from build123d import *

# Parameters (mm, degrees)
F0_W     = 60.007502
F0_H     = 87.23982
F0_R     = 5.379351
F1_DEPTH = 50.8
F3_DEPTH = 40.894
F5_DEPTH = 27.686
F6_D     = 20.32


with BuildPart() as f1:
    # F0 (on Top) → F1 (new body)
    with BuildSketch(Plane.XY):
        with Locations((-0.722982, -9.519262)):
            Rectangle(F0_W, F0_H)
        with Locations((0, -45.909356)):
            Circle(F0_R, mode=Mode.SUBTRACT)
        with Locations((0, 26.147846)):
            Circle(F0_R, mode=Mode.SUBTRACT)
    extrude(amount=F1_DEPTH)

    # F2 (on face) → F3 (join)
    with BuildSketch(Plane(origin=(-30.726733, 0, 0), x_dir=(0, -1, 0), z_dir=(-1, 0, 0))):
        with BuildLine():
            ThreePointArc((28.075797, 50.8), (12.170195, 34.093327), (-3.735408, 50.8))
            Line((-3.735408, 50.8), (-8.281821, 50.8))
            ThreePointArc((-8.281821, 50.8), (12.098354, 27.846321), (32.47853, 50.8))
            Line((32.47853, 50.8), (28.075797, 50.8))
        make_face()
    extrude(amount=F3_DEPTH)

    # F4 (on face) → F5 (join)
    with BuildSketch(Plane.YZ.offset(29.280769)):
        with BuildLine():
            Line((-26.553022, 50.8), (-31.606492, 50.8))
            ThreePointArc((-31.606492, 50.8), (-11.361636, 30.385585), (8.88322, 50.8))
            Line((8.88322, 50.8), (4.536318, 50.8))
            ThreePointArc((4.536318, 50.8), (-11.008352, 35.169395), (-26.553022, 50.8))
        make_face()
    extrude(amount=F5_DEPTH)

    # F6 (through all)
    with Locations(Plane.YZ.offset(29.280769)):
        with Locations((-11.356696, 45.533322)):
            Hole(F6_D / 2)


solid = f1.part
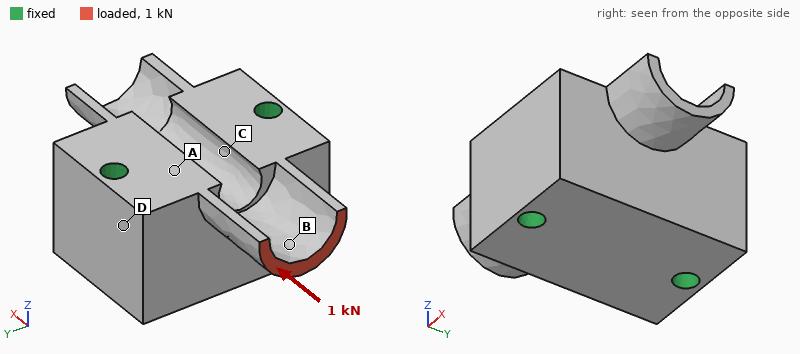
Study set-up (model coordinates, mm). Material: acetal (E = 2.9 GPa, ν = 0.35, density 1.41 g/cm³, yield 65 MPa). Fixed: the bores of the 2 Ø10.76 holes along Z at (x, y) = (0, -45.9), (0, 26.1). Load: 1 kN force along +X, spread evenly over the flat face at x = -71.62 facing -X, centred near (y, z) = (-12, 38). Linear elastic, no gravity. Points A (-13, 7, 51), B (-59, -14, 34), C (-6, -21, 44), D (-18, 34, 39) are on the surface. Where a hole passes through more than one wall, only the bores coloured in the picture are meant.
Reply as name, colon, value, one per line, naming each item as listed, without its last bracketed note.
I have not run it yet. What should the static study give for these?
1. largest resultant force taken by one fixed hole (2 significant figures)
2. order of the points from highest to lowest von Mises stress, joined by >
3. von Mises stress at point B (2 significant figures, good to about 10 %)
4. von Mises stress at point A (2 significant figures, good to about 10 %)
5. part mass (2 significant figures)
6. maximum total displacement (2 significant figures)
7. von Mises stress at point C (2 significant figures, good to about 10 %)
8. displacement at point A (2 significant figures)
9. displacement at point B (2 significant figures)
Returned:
largest resultant force taken by one fixed hole: 550 N
order of the points from highest to lowest von Mises stress, joined by >: B > A > C > D
von Mises stress at point B: 3.0 MPa
von Mises stress at point A: 0.97 MPa
part mass: 370 g
maximum total displacement: 61 µm
von Mises stress at point C: 0.53 MPa
displacement at point A: 9.9 µm
displacement at point B: 43 µm
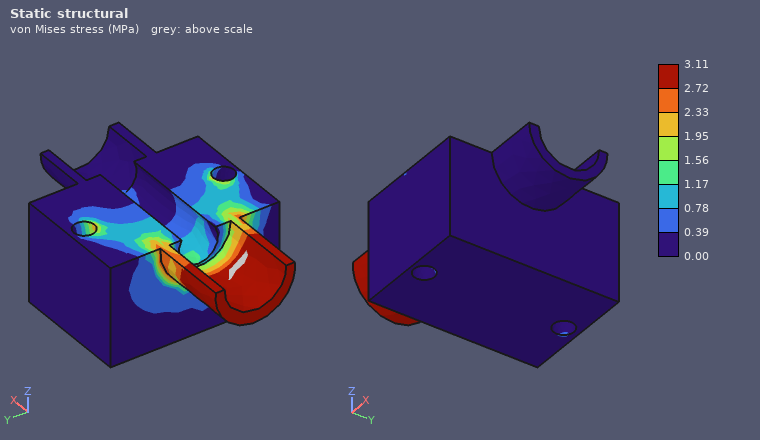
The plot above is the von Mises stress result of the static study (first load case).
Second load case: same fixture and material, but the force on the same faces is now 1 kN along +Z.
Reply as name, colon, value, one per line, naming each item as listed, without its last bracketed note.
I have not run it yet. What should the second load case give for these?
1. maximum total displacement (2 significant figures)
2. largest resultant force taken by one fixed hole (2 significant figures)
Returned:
maximum total displacement: 1.4 mm
largest resultant force taken by one fixed hole: 530 N
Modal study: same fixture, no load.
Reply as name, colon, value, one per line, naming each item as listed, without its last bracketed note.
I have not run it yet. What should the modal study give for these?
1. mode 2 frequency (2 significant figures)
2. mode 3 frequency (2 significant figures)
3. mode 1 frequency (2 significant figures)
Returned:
mode 2 frequency: 1800 Hz
mode 3 frequency: 2200 Hz
mode 1 frequency: 1500 Hz
